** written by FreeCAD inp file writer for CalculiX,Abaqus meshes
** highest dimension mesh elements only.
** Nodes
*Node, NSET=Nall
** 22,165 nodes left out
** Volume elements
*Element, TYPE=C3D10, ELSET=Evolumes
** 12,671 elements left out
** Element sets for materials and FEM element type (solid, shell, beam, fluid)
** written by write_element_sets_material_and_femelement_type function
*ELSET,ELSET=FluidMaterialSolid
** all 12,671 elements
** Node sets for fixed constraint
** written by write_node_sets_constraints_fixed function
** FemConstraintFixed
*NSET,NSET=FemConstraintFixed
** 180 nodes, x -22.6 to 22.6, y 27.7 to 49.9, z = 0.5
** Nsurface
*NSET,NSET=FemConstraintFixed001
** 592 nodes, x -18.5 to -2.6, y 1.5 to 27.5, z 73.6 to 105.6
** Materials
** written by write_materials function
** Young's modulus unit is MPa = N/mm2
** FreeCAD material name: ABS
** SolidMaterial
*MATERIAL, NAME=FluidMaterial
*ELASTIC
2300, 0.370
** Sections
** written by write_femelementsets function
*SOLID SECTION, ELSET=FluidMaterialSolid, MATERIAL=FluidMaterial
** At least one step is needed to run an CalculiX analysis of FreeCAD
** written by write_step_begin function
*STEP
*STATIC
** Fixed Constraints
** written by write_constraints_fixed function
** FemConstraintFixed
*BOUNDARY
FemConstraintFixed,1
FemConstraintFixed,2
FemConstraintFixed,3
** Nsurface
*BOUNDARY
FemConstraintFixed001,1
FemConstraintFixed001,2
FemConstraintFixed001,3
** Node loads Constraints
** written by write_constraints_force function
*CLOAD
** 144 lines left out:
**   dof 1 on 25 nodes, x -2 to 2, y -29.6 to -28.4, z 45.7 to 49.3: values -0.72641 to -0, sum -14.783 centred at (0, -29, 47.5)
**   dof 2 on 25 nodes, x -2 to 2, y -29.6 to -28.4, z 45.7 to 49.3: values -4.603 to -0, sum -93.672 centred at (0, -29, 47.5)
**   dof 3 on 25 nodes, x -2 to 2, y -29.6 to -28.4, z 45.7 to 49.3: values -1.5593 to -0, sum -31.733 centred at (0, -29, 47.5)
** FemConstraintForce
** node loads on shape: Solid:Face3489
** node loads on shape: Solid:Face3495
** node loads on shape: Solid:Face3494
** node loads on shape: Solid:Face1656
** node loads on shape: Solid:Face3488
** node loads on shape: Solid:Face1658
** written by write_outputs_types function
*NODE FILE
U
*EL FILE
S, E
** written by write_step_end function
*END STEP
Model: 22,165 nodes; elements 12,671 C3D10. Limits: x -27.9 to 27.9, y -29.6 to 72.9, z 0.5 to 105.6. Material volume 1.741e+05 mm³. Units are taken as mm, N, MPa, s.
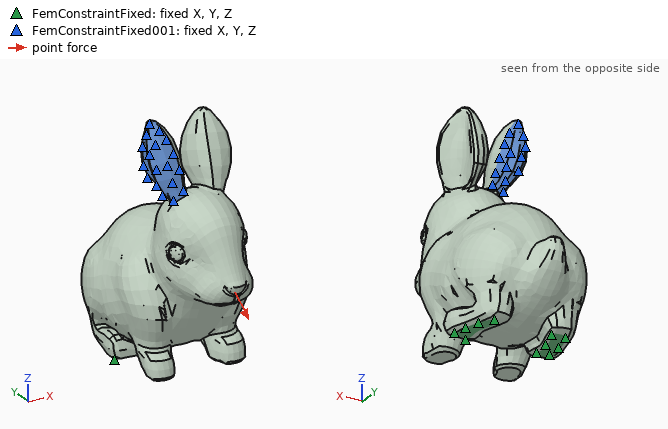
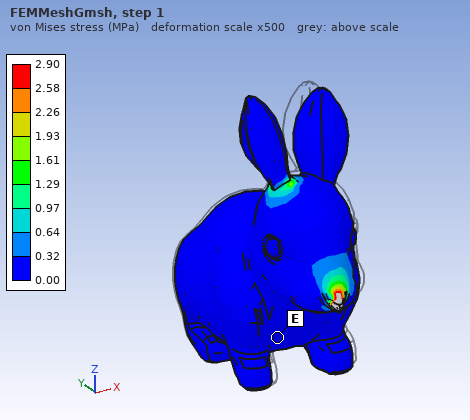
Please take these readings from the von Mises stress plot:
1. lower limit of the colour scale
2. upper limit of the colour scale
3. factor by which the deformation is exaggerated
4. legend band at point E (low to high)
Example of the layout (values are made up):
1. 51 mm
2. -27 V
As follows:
1. 0.00 MPa
2. 2.90 MPa
3. 500
4. 0.00 to 0.32 MPa
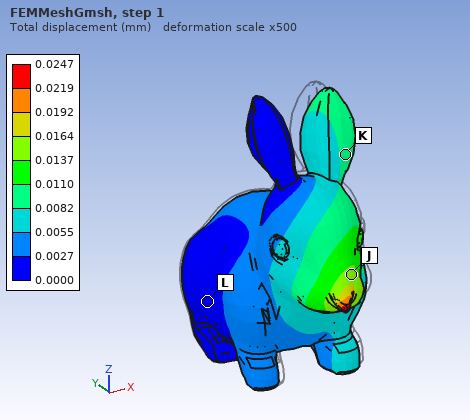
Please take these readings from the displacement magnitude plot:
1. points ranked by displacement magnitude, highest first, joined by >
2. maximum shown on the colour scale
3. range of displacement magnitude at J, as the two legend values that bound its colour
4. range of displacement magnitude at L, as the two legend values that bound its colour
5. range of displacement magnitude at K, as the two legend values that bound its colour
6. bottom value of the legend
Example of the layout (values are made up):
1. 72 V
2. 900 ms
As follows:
1. J > K > L
2. 0.0247 mm
3. 0.0137 to 0.0164 mm
4. 0.0000 to 0.0027 mm
5. 0.0082 to 0.0110 mm
6. 0.0000 mm
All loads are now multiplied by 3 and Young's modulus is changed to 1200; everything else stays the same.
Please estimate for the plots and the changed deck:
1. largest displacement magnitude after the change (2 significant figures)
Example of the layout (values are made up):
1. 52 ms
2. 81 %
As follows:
1. 0.14 mm
